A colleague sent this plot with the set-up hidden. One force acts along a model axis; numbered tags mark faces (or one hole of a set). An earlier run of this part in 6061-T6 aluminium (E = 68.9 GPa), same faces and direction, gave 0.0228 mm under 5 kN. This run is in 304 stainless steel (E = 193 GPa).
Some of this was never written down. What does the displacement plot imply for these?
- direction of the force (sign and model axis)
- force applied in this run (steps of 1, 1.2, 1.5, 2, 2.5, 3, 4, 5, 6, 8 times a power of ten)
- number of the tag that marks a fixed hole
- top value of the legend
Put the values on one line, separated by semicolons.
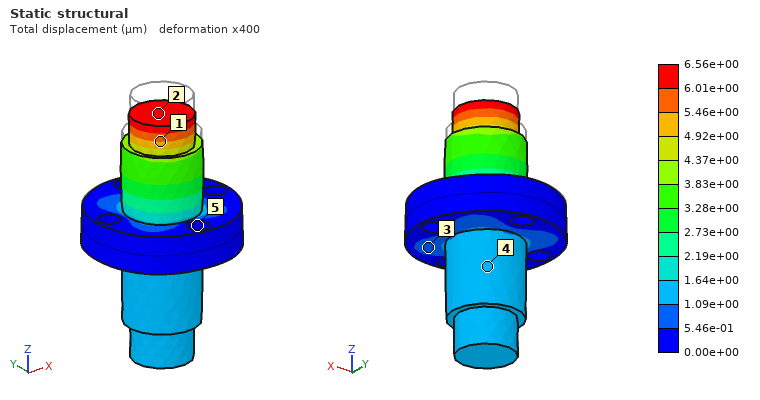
-Z; 4 kN; 5; 6.56e+00 µm
